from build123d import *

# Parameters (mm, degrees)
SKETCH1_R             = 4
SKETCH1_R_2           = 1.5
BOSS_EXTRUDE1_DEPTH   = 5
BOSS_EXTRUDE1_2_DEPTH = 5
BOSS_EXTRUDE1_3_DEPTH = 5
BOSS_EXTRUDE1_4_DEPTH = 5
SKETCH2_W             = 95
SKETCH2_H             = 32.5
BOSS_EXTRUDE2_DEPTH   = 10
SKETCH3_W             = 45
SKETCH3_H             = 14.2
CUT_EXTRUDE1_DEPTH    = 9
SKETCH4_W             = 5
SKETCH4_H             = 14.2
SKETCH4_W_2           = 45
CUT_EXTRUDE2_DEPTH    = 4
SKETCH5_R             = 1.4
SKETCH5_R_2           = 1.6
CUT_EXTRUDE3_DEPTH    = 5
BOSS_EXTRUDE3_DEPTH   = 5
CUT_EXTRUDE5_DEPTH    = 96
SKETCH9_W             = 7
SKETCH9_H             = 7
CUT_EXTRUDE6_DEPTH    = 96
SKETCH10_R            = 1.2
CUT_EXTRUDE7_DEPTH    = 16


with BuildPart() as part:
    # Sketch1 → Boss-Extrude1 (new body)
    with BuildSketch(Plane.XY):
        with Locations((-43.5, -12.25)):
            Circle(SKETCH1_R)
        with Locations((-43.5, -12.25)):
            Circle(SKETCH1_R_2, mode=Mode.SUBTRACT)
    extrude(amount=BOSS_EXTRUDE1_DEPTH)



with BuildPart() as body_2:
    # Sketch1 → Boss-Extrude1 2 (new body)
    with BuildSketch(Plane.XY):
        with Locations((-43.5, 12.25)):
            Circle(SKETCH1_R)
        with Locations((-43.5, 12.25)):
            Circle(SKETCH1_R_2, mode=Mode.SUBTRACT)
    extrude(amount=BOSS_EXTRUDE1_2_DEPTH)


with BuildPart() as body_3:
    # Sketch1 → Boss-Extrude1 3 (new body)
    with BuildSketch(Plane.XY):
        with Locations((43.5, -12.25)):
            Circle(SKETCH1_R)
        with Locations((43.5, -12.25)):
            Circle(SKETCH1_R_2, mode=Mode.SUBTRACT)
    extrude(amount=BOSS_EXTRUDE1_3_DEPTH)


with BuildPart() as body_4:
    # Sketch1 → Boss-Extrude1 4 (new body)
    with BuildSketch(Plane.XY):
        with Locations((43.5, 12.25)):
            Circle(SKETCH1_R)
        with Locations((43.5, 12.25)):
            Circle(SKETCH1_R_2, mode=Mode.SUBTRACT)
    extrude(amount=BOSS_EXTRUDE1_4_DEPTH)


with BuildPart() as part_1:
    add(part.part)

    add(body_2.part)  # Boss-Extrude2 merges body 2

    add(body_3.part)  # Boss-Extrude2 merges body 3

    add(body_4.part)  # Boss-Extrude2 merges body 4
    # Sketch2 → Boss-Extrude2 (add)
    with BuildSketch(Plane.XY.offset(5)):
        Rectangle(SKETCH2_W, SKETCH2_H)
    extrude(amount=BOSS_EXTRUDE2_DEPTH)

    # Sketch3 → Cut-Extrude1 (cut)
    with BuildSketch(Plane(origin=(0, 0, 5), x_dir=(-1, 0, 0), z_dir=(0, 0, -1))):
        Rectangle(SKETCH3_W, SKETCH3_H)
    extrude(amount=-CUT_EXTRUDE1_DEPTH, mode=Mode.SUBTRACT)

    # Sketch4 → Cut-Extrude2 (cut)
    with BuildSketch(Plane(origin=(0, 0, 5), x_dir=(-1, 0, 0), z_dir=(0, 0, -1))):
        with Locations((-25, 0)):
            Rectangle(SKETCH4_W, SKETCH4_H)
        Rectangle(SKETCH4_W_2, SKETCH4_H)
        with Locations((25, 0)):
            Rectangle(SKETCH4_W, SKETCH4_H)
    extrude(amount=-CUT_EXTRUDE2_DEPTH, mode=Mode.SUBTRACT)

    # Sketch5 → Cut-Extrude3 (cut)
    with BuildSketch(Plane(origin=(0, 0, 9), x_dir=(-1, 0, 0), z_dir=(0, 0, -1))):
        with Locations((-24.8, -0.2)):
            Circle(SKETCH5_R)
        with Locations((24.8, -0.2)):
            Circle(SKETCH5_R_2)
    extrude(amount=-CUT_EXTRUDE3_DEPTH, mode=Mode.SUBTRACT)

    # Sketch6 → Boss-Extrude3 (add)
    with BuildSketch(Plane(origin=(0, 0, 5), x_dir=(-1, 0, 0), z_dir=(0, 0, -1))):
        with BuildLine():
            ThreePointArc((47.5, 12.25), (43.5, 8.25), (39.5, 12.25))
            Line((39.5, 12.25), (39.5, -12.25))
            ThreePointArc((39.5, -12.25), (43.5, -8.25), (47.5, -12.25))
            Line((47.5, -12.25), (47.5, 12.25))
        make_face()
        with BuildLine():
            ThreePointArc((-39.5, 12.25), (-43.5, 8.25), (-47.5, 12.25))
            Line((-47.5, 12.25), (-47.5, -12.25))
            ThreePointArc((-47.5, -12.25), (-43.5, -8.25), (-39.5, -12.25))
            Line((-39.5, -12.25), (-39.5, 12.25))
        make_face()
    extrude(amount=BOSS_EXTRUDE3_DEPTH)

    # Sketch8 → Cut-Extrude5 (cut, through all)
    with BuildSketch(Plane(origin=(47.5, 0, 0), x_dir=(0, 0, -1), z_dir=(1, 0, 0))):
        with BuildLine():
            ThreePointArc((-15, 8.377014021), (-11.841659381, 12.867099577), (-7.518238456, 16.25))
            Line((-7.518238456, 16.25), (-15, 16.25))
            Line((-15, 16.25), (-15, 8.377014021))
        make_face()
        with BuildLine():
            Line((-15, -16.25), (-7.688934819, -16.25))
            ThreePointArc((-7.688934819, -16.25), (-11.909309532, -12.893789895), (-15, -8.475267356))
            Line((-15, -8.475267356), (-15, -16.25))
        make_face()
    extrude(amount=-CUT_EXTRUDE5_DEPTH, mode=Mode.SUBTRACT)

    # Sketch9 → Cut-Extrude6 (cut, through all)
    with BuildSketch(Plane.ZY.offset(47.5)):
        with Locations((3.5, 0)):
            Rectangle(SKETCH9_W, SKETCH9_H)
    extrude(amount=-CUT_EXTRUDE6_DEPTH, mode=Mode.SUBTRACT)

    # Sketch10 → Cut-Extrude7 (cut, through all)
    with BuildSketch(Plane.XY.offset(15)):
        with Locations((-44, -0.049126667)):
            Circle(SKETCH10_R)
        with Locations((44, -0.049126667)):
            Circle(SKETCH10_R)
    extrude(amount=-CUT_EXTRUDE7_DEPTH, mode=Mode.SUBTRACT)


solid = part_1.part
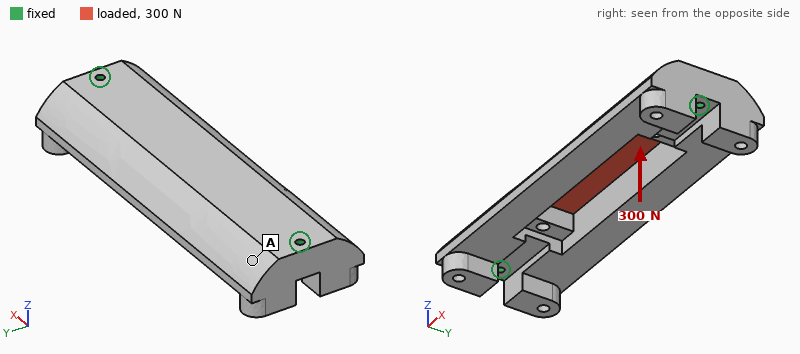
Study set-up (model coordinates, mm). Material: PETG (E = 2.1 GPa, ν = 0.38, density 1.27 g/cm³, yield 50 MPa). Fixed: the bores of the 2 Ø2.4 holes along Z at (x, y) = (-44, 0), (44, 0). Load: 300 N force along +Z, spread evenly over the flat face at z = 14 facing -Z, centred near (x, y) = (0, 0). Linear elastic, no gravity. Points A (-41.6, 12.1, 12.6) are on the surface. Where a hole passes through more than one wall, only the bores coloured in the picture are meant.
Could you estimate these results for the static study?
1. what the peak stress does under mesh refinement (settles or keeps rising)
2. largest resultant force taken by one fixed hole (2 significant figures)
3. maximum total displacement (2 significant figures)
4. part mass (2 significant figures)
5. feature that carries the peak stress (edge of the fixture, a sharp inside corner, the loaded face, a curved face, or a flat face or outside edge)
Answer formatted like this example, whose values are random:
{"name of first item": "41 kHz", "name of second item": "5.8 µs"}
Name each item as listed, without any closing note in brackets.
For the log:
{"what the peak stress does under mesh refinement": "keeps rising", "largest resultant force taken by one fixed hole": "180 N", "maximum total displacement": "0.75 mm", "part mass": "27 g", "feature that carries the peak stress": "edge of the fixture"}
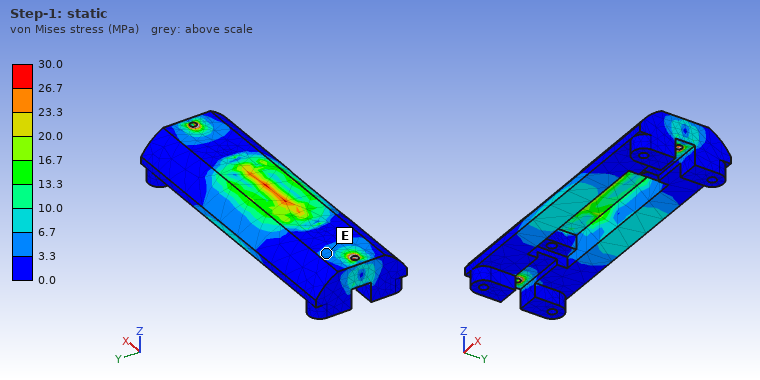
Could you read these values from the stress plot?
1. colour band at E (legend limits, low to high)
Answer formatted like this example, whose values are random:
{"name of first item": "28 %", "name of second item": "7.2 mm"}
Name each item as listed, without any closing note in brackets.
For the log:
{"colour band at E": "3.3 to 6.7 MPa"}
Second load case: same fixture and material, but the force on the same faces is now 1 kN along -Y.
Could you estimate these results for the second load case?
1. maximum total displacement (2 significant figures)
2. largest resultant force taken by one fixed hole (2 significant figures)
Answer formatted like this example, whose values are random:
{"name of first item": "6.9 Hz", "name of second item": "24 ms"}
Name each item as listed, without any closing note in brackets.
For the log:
{"maximum total displacement": "0.77 mm", "largest resultant force taken by one fixed hole": "500 N"}
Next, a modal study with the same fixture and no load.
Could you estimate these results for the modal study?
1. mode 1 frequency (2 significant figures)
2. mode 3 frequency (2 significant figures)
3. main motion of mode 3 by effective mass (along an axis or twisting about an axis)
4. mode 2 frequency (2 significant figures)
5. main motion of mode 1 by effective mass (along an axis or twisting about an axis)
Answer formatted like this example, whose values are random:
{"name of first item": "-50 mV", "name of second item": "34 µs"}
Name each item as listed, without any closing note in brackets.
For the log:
{"mode 1 frequency": "1200 Hz", "mode 3 frequency": "2200 Hz", "main motion of mode 3 by effective mass": "along Y", "mode 2 frequency": "1500 Hz", "main motion of mode 1 by effective mass": "along Z"}
